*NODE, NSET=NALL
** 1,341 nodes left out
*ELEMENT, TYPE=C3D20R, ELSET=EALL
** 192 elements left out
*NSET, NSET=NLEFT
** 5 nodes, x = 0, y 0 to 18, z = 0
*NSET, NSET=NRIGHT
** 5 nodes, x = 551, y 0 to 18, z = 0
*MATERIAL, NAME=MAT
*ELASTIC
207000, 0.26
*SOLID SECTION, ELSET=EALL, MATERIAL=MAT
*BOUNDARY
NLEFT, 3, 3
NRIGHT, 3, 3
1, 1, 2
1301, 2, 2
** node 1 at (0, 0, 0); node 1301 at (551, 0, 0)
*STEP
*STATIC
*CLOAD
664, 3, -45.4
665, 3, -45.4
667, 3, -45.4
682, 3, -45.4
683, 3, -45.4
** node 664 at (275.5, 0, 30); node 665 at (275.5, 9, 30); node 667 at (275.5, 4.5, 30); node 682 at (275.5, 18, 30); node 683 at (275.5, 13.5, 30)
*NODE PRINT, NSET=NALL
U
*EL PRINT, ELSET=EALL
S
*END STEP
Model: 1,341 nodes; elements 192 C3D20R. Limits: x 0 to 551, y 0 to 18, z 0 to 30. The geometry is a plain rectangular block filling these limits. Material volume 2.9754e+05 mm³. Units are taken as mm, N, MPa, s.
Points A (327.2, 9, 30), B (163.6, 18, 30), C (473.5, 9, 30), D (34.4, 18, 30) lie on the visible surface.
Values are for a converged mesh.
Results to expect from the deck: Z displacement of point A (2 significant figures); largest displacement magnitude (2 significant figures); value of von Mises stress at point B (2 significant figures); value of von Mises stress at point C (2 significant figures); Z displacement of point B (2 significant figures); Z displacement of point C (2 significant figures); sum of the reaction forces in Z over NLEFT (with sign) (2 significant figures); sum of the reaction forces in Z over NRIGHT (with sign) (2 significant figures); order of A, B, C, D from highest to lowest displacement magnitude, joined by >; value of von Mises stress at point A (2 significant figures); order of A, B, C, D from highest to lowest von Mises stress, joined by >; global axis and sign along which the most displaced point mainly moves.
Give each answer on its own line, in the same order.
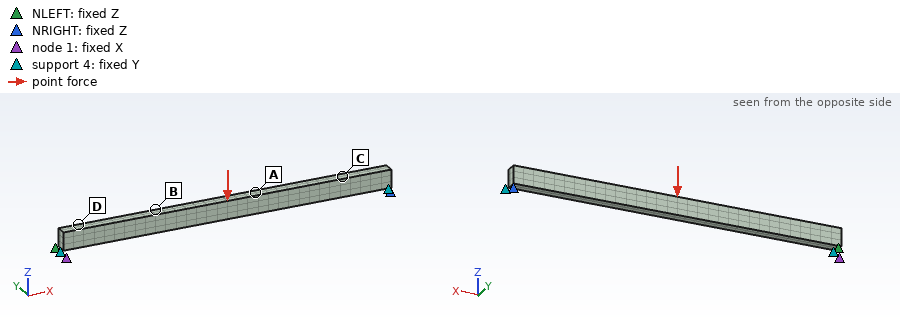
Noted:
-0.090 mm
0.096 mm
6.9 MPa
3.3 MPa
-0.075 mm
-0.039 mm
110 N
110 N
A > B > C > D
9.4 MPa
A > B > C > D
-Z
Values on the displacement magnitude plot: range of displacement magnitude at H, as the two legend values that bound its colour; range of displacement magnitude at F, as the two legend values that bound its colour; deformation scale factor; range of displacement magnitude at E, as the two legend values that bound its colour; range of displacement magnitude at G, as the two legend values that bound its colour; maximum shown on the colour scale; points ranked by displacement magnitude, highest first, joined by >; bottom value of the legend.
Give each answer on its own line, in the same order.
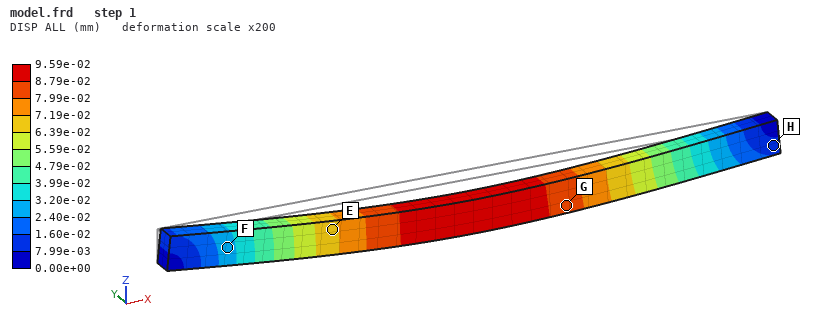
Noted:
7.99e-03 to 1.60e-02 mm
2.40e-02 to 3.20e-02 mm
200
6.39e-02 to 7.19e-02 mm
7.99e-02 to 8.79e-02 mm
9.59e-02 mm
G > E > F > H
0.00e+00 mm
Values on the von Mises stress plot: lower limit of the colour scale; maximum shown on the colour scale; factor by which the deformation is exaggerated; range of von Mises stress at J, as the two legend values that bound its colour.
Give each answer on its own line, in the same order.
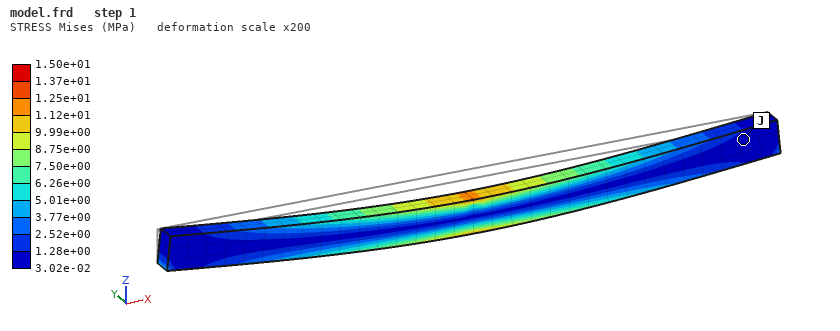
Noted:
3.02e-02 MPa
1.50e+01 MPa
200
3.02e-02 to 1.28e+00 MPa
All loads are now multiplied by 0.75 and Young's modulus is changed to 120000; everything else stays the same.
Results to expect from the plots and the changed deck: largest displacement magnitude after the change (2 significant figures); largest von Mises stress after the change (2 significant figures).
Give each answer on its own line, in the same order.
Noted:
0.12 mm
11 MPa
